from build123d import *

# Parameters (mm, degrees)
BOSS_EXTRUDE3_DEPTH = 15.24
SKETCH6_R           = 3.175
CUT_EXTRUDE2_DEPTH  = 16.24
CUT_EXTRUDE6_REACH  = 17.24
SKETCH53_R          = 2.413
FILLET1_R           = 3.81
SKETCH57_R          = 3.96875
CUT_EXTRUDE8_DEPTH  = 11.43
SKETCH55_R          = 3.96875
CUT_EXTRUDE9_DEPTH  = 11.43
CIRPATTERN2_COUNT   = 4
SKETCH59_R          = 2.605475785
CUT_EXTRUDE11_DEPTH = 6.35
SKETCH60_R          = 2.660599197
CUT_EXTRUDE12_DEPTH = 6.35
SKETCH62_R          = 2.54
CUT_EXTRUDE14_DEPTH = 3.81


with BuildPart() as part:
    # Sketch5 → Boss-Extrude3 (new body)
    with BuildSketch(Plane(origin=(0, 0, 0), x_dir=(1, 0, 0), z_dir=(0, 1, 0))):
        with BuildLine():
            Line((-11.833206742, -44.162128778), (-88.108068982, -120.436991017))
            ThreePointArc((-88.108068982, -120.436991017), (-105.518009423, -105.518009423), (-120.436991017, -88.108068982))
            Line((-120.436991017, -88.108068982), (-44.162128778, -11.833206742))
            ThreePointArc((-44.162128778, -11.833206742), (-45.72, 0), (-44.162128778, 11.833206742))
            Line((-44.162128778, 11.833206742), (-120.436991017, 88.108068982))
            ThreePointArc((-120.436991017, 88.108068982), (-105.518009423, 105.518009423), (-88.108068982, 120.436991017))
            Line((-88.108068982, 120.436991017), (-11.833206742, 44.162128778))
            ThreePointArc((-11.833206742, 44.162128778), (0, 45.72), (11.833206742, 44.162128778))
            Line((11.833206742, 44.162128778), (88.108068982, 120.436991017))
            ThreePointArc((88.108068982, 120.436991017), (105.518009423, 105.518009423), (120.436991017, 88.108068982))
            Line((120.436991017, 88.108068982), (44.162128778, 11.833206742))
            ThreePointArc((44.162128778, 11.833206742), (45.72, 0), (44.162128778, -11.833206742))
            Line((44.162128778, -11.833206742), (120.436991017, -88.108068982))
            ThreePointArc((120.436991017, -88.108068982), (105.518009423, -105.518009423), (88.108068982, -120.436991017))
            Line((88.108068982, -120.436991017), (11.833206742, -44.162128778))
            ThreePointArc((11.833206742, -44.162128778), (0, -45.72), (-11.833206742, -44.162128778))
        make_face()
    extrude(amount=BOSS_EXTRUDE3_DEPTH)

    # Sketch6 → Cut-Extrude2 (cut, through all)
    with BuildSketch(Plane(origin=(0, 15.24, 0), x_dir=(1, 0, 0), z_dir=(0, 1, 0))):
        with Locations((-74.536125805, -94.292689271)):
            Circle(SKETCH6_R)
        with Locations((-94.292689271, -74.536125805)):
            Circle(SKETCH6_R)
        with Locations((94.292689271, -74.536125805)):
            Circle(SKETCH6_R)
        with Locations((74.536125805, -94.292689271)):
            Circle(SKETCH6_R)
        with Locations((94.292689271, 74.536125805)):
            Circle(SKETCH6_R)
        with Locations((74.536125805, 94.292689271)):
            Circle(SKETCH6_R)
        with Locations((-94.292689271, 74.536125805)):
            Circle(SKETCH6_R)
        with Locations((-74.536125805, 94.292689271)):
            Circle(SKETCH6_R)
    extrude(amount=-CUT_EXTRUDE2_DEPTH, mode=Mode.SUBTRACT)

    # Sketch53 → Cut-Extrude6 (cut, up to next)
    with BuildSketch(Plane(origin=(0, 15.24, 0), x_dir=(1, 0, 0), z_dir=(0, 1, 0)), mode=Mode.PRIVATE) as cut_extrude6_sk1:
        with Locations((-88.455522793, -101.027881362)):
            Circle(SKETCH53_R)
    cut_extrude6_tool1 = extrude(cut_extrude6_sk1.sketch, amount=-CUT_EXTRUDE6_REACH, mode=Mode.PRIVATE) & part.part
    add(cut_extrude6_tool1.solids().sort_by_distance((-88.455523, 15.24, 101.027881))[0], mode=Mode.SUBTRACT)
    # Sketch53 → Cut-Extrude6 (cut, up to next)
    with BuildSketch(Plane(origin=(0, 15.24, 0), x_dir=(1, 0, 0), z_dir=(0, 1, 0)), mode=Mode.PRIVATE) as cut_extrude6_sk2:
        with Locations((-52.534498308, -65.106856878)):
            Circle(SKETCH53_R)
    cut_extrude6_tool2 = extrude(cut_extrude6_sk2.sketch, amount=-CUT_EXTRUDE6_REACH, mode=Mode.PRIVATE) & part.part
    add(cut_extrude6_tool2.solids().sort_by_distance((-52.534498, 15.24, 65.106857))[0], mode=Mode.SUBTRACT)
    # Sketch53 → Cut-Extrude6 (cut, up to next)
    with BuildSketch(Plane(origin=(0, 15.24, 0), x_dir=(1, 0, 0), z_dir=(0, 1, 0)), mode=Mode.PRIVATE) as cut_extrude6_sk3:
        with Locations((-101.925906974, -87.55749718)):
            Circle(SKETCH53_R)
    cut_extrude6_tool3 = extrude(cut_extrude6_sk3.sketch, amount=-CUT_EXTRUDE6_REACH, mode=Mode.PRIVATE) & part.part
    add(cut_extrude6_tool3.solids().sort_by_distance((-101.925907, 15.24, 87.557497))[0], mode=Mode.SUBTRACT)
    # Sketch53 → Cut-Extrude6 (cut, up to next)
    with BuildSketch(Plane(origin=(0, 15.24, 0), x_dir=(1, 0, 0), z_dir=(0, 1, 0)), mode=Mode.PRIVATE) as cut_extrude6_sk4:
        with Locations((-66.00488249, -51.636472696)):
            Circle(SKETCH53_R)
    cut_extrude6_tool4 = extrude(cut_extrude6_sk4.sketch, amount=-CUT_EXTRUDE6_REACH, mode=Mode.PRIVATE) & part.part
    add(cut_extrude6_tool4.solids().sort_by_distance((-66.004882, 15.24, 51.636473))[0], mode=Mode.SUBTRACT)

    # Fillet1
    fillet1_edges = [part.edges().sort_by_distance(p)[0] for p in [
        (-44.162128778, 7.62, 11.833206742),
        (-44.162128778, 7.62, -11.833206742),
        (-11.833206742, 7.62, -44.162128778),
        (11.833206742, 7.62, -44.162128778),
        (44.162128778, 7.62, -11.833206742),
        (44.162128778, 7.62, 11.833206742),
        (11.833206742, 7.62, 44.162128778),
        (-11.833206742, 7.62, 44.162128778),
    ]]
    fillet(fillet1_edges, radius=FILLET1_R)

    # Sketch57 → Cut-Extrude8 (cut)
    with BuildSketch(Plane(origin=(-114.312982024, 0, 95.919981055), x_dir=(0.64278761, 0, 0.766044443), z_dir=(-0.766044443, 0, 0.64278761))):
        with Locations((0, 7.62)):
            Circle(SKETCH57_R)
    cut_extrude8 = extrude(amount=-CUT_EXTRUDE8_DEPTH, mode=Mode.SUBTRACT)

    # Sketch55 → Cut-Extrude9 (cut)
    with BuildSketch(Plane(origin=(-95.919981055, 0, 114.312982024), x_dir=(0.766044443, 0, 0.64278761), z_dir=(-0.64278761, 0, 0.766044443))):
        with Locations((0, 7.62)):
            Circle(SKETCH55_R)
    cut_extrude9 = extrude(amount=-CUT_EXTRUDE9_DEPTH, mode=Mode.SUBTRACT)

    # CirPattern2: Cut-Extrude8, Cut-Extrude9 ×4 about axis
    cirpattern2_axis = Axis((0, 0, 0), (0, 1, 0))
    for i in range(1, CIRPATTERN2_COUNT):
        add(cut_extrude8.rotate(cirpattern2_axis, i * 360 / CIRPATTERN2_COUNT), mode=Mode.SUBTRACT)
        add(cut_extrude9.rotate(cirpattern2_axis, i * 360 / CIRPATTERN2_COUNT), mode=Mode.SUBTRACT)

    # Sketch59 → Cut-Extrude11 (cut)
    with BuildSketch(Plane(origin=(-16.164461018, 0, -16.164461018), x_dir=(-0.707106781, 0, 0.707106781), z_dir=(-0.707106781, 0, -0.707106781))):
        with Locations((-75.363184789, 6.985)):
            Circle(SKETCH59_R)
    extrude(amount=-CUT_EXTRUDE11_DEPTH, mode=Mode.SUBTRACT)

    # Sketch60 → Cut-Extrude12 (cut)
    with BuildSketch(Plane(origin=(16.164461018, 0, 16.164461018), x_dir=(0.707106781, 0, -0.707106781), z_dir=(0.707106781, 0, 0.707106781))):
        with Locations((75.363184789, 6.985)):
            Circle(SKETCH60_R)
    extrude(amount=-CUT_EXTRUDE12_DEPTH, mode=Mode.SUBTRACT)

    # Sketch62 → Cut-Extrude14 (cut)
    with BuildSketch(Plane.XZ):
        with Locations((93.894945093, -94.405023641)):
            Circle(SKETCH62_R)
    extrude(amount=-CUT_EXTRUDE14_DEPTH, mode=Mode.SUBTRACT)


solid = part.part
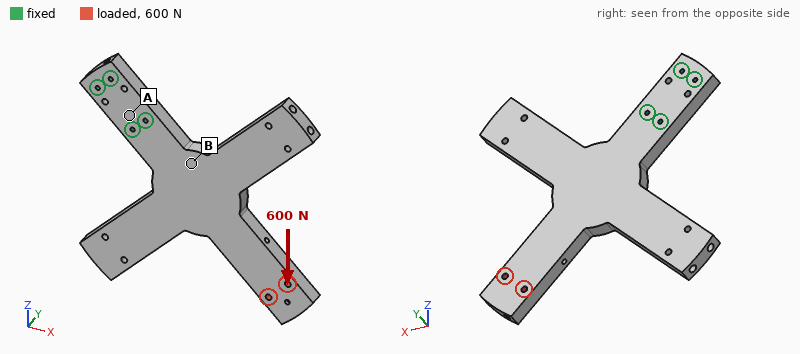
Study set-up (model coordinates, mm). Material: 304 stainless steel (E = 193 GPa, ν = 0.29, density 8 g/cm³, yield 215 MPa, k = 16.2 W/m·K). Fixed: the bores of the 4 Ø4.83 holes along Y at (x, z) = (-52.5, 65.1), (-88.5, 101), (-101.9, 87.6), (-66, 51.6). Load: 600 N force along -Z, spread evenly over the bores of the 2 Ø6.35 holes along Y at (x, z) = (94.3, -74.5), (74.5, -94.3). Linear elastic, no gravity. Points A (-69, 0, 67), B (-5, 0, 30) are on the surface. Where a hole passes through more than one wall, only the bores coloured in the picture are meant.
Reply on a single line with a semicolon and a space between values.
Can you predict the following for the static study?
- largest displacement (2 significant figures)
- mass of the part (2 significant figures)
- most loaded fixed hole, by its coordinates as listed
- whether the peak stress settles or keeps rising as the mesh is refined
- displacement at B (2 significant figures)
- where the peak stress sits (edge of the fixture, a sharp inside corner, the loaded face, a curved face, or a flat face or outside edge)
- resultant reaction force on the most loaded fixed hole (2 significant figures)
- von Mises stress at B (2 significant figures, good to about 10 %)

55 µm; 3.1 kg; (-52.5, 65.1); keeps rising; 8.9 µm; edge of the fixture; 2.9 kN; 5.4 MPa
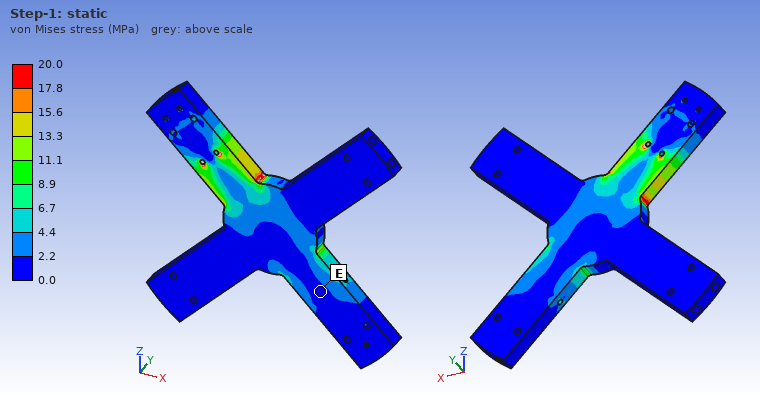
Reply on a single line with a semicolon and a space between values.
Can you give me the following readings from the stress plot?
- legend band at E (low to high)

0.0 to 2.2 MPa
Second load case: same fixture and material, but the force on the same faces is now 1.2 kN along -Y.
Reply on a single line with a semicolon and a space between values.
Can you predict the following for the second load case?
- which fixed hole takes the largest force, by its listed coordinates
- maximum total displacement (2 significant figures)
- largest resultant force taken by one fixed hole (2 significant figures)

(-52.5, 65.1); 1.4 mm; 1.2 kN
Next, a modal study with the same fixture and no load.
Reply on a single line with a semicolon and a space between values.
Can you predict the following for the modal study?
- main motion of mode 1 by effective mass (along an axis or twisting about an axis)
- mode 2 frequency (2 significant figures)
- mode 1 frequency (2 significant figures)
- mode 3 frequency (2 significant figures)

along Y; 320 Hz; 220 Hz; 500 Hz
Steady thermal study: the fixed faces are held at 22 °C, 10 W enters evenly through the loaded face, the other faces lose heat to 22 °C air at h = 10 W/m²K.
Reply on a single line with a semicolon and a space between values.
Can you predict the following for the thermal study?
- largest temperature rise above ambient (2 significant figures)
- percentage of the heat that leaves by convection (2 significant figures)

58 K; 88 %
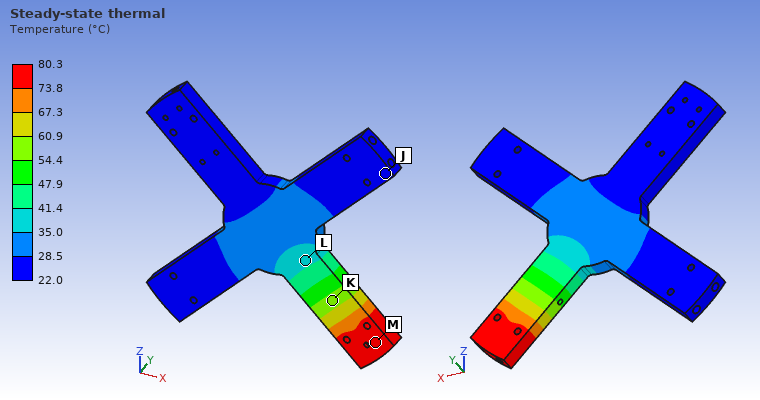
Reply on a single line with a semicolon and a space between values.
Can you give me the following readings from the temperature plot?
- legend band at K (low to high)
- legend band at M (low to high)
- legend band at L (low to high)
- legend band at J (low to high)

54.4 to 60.9 °C; 73.8 to 80.3 °C; 35.0 to 41.4 °C; 22.0 to 28.5 °C
